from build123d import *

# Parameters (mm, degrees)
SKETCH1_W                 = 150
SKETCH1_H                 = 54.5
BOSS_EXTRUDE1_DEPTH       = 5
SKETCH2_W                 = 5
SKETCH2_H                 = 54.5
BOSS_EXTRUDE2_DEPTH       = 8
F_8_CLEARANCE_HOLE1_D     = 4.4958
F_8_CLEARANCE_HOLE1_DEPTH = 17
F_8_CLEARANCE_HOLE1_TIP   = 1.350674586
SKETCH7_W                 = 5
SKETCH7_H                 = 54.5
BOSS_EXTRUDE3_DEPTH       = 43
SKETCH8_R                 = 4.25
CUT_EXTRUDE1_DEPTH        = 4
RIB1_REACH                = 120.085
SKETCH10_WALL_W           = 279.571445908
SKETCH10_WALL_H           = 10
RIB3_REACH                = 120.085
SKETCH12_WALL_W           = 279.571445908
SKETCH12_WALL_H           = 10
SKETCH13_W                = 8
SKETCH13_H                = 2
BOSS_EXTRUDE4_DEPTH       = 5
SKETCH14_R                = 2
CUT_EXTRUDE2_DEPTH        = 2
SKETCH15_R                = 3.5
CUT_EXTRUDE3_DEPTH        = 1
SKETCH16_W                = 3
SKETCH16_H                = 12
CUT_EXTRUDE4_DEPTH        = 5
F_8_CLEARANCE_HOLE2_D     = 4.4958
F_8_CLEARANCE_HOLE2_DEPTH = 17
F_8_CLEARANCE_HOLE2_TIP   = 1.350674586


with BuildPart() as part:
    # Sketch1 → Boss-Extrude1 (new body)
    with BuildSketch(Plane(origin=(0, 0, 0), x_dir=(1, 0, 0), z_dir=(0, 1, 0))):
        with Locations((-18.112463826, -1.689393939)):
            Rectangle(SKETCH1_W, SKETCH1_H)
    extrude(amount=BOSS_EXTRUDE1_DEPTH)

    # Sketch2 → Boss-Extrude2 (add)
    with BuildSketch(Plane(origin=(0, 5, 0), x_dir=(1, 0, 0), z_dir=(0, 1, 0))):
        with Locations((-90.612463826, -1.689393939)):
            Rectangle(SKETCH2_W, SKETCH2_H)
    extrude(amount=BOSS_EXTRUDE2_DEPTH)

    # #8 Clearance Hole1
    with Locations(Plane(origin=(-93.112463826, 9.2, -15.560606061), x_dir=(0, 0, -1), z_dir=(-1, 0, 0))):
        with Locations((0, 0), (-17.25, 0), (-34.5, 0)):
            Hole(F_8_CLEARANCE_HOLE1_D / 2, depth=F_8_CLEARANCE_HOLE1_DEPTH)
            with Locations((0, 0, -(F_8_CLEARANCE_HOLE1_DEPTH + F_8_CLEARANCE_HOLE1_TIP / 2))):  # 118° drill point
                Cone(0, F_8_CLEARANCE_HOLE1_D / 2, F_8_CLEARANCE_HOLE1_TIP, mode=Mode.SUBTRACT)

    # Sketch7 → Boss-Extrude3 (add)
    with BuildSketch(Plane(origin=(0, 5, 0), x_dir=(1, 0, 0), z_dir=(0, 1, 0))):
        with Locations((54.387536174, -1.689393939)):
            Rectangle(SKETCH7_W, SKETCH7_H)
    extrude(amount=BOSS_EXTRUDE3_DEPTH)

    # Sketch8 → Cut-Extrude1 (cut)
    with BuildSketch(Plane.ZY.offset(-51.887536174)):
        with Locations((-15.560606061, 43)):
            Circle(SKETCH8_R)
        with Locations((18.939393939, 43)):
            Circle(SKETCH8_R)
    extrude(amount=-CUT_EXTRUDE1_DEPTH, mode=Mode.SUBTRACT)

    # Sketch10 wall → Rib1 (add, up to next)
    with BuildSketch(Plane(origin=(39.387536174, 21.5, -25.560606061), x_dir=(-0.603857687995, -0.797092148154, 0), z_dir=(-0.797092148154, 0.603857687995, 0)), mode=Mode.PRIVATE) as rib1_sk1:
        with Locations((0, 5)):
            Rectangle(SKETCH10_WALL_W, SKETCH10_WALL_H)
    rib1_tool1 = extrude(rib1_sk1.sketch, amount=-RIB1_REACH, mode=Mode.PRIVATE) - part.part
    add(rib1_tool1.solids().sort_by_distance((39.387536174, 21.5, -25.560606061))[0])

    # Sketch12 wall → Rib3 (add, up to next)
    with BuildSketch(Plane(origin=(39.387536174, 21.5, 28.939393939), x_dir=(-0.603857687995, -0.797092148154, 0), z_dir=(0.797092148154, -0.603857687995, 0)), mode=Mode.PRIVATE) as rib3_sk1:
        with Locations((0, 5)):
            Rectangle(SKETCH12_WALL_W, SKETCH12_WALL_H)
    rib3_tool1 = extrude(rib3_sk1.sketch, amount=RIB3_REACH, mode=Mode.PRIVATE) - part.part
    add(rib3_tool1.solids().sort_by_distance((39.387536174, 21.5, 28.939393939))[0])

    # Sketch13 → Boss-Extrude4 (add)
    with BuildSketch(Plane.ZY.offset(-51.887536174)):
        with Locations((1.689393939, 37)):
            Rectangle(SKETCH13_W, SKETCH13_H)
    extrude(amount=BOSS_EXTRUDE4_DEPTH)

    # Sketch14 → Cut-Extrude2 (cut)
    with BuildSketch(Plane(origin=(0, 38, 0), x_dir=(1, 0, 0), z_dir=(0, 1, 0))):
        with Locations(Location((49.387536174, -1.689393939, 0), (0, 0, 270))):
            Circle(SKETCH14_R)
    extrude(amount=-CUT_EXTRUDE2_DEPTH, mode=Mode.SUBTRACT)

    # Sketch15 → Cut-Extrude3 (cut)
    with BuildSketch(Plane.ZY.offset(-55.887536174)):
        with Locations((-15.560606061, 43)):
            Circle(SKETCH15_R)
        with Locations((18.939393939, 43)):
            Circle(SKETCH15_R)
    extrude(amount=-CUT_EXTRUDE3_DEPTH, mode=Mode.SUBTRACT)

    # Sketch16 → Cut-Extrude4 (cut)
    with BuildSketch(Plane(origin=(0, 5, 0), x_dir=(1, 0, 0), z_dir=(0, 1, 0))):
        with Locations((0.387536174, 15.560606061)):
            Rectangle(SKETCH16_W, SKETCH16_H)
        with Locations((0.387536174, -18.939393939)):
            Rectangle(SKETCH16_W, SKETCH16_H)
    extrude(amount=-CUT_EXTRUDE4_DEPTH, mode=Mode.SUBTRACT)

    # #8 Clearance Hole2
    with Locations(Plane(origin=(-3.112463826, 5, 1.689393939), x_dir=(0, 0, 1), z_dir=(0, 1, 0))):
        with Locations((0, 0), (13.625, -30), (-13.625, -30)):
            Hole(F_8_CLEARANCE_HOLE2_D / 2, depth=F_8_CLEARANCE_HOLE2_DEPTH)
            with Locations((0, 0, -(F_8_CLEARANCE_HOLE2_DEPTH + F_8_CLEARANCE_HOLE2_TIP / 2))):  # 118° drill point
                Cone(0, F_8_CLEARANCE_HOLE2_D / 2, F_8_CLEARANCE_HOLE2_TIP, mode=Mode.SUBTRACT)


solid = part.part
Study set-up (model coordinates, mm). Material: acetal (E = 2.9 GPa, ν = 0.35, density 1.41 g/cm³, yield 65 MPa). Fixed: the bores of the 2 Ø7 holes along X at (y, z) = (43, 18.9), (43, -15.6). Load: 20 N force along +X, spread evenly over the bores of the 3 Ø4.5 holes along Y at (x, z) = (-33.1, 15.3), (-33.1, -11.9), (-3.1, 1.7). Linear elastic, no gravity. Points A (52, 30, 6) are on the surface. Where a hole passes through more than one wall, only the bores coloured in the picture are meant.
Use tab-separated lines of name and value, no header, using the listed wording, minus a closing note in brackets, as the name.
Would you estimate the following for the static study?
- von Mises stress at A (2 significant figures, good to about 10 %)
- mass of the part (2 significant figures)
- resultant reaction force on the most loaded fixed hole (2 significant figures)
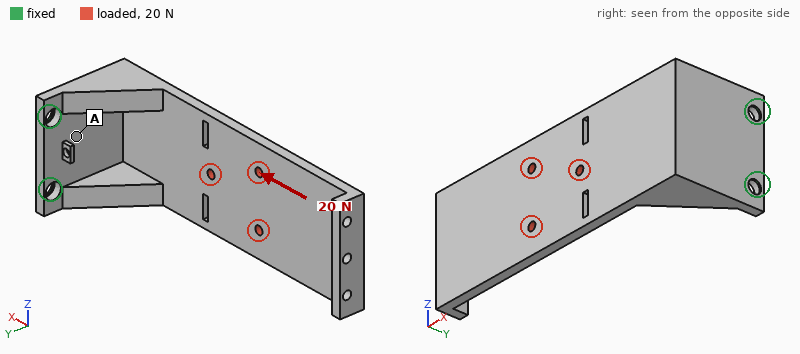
von Mises stress at A	1.4 MPa
mass of the part	87 g
resultant reaction force on the most loaded fixed hole	11 N
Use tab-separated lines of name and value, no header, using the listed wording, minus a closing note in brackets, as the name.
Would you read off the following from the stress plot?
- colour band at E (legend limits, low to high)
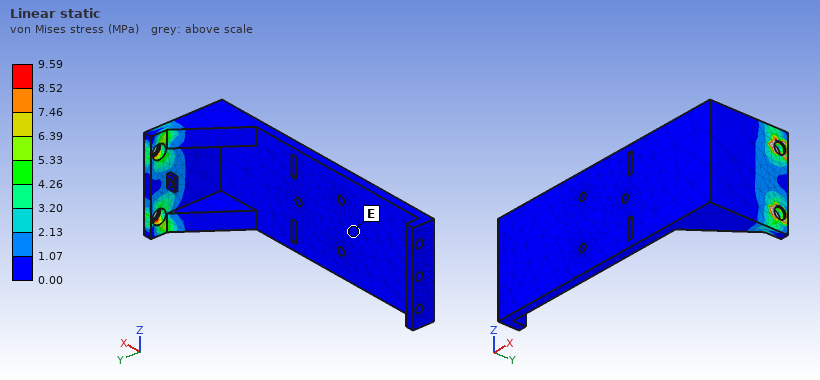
colour band at E	0.00 to 1.07 MPa
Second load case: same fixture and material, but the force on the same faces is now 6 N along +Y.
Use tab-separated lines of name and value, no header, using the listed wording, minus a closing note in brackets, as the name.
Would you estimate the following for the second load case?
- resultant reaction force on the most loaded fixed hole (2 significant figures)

resultant reaction force on the most loaded fixed hole	6.6 N
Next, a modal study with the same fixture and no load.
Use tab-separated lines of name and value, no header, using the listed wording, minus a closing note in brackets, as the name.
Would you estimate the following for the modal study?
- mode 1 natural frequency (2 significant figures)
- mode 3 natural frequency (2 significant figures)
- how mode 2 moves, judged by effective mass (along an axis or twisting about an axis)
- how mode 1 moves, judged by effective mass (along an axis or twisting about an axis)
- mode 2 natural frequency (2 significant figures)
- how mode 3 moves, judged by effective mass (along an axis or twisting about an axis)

mode 1 natural frequency	41 Hz
mode 3 natural frequency	160 Hz
how mode 2 moves, judged by effective mass	along Z
how mode 1 moves, judged by effective mass	along Y
mode 2 natural frequency	110 Hz
how mode 3 moves, judged by effective mass	along X
